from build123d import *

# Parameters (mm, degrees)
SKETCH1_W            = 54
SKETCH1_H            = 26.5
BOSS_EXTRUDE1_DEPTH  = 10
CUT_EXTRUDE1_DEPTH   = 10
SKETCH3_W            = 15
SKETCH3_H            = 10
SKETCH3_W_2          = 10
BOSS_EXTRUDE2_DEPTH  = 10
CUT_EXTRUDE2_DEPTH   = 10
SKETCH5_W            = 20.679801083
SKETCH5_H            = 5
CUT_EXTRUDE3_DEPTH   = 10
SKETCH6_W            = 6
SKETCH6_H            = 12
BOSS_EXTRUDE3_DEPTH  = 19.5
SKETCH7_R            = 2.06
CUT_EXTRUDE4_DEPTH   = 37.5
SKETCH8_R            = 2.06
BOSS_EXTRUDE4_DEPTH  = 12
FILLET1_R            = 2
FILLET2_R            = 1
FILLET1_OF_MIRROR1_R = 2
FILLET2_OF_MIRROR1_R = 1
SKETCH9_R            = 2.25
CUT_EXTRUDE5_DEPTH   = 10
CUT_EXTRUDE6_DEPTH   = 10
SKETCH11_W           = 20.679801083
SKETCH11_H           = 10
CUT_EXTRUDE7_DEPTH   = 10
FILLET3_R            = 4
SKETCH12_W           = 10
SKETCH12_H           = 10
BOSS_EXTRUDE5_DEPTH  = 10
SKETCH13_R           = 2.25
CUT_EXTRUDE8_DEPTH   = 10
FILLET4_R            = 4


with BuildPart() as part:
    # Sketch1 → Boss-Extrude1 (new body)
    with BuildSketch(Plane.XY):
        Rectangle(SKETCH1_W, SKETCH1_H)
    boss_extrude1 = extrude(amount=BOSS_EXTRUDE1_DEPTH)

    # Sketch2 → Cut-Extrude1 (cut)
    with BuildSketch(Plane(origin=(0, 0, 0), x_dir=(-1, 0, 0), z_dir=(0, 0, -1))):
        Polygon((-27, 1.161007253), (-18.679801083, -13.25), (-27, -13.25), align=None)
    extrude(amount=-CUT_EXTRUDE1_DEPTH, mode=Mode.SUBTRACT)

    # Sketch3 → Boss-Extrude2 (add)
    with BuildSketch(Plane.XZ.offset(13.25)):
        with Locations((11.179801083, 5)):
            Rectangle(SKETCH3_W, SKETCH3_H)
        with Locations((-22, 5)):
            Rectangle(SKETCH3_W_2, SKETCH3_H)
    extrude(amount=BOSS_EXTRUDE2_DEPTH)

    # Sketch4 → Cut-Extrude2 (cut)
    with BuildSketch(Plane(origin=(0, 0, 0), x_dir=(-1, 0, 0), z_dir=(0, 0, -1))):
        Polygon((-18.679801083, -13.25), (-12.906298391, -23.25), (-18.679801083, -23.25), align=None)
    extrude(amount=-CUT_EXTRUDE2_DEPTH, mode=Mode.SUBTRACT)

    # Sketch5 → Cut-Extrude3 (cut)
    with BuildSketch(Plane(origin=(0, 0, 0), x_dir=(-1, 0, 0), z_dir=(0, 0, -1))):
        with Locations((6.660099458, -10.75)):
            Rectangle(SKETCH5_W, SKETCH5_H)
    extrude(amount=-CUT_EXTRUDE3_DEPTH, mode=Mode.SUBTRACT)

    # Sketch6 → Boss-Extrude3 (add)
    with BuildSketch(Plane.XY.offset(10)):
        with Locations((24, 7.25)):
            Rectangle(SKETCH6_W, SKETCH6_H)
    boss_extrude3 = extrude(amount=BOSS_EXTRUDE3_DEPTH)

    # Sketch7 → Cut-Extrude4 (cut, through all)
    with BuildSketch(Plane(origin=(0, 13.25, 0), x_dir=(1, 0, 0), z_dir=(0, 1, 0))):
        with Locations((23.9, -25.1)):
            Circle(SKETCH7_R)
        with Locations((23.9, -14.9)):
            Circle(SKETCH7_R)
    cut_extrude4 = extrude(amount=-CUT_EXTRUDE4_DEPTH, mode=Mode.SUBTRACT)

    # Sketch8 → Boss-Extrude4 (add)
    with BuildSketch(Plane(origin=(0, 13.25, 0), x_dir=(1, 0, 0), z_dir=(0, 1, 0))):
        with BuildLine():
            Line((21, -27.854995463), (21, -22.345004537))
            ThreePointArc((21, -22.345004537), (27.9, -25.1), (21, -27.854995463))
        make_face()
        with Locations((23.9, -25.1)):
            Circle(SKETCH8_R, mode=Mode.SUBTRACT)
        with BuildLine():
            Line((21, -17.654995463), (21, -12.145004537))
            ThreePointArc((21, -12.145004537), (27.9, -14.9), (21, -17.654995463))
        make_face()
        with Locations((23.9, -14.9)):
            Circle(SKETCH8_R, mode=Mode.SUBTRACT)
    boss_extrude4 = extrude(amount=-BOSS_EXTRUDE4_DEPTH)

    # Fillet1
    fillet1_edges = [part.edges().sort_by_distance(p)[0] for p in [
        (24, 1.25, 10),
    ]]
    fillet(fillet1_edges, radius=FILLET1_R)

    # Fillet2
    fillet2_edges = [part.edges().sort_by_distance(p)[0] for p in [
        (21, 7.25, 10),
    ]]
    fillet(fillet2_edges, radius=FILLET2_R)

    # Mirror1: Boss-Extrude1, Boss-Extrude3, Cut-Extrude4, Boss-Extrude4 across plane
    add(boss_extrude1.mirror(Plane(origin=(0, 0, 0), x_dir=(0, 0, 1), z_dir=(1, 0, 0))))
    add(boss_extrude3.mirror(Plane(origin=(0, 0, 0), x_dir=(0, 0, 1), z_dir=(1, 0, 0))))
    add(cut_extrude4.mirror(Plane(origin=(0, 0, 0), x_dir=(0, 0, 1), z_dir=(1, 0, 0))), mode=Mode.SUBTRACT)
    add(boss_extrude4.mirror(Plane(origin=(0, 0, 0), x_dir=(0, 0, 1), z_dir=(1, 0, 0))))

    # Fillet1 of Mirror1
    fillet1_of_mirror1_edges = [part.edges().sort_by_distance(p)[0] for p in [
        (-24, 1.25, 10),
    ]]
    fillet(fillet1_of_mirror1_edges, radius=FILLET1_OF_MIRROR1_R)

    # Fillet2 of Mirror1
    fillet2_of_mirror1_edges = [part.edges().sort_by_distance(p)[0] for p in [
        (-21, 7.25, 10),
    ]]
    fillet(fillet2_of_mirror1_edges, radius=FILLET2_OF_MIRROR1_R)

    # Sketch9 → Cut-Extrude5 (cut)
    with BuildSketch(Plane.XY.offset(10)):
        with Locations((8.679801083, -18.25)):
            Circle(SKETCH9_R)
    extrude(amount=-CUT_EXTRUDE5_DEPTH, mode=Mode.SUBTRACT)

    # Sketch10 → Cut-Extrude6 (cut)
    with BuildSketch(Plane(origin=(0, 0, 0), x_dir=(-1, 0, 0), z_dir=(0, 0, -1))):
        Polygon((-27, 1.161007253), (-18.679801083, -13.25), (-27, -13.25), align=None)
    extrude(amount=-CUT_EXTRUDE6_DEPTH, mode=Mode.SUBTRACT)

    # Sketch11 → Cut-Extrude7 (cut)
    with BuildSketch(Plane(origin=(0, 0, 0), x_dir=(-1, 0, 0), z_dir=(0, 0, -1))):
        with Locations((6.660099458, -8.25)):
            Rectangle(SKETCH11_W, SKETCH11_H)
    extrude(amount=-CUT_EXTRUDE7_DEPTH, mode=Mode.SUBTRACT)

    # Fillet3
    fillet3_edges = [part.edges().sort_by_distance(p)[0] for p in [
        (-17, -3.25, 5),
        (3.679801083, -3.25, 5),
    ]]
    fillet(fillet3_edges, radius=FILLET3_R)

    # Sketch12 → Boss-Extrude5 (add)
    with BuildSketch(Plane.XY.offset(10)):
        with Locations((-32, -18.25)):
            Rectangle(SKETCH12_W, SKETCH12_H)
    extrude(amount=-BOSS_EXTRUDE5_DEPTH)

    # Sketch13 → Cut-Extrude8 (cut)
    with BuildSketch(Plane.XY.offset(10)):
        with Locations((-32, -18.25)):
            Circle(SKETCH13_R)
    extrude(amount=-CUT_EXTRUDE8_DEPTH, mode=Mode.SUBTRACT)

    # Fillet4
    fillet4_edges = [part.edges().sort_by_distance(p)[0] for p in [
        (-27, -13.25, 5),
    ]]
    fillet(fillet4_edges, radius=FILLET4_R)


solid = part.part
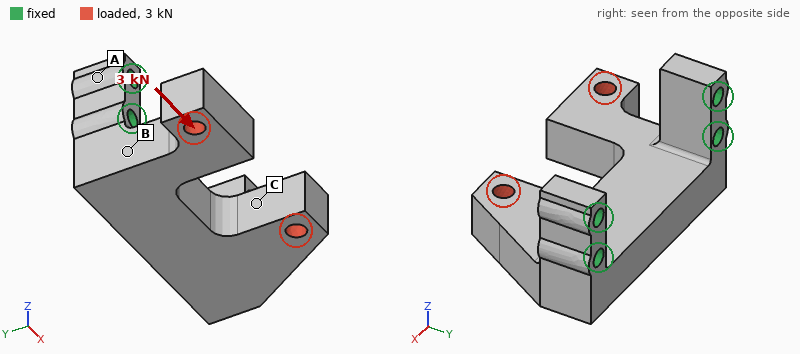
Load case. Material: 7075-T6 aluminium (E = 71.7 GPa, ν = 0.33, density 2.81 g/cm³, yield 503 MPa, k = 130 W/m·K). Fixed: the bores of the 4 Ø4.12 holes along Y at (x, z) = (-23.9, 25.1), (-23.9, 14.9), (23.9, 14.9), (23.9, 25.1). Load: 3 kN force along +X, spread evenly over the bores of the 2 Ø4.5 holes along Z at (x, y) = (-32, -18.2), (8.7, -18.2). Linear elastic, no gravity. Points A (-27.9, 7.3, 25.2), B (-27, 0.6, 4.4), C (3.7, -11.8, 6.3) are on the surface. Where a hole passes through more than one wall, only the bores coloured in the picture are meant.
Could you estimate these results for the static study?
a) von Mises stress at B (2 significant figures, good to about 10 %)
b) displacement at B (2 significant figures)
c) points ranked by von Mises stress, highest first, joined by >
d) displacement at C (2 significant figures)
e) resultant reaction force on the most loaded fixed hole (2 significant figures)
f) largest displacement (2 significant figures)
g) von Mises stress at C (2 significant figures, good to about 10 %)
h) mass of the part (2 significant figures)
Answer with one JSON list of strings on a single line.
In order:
["81 MPa", "0.022 mm", "B > C > A", "0.024 mm", "2.2 kN", "0.15 mm", "28 MPa", "48 g"]
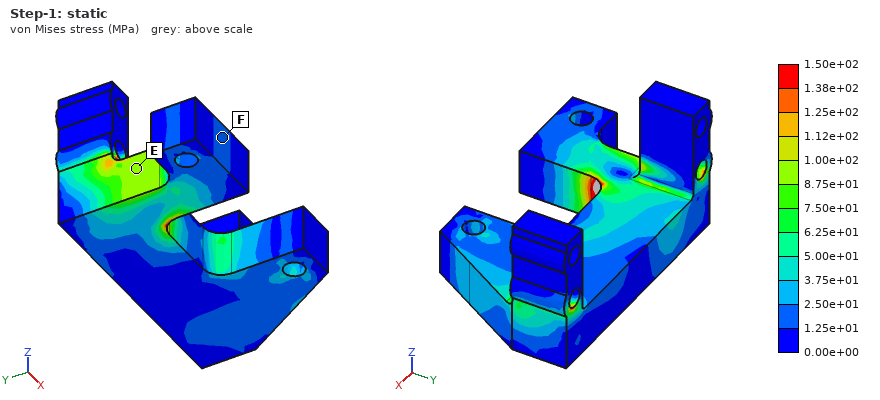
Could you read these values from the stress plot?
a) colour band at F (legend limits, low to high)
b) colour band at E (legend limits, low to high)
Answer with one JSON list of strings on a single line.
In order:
["1.25e+01 to 2.50e+01 MPa", "8.75e+01 to 1.00e+02 MPa"]
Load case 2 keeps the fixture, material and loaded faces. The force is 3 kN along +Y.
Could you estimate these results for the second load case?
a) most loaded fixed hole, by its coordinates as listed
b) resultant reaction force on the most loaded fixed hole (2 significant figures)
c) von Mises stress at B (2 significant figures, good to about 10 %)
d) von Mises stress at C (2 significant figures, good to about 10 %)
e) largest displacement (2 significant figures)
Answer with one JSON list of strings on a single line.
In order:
["(-23.9, 14.9)", "2.2 kN", "64 MPa", "21 MPa", "0.12 mm"]
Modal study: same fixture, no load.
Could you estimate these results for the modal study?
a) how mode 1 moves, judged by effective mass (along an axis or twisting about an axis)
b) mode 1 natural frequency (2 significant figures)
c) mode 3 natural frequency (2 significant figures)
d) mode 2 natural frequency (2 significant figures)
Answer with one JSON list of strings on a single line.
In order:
["along Z", "5500 Hz", "7900 Hz", "6900 Hz"]
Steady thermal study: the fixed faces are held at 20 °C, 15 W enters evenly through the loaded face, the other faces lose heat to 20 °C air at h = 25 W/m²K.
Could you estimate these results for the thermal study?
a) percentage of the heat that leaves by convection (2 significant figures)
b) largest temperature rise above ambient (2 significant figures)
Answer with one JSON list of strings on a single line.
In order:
["7.4 %", "20 K"]
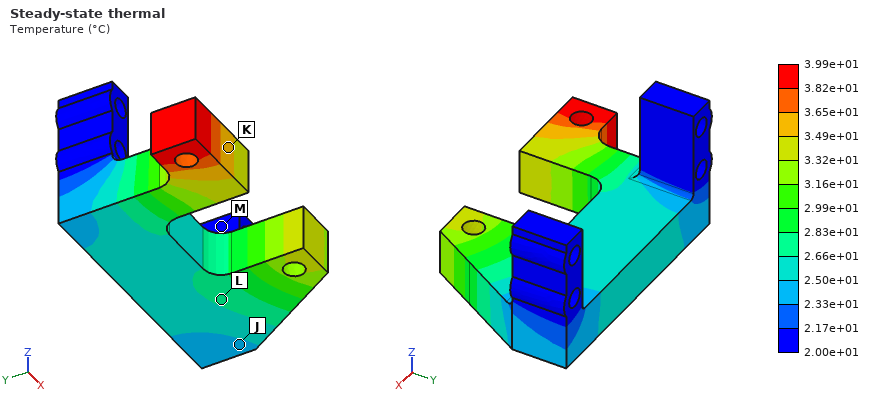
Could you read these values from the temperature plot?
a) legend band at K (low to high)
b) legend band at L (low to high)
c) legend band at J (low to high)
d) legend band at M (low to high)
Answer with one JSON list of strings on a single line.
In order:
["3.49e+01 to 3.65e+01 °C", "2.66e+01 to 2.83e+01 °C", "2.33e+01 to 2.50e+01 °C", "2.00e+01 to 2.17e+01 °C"]
